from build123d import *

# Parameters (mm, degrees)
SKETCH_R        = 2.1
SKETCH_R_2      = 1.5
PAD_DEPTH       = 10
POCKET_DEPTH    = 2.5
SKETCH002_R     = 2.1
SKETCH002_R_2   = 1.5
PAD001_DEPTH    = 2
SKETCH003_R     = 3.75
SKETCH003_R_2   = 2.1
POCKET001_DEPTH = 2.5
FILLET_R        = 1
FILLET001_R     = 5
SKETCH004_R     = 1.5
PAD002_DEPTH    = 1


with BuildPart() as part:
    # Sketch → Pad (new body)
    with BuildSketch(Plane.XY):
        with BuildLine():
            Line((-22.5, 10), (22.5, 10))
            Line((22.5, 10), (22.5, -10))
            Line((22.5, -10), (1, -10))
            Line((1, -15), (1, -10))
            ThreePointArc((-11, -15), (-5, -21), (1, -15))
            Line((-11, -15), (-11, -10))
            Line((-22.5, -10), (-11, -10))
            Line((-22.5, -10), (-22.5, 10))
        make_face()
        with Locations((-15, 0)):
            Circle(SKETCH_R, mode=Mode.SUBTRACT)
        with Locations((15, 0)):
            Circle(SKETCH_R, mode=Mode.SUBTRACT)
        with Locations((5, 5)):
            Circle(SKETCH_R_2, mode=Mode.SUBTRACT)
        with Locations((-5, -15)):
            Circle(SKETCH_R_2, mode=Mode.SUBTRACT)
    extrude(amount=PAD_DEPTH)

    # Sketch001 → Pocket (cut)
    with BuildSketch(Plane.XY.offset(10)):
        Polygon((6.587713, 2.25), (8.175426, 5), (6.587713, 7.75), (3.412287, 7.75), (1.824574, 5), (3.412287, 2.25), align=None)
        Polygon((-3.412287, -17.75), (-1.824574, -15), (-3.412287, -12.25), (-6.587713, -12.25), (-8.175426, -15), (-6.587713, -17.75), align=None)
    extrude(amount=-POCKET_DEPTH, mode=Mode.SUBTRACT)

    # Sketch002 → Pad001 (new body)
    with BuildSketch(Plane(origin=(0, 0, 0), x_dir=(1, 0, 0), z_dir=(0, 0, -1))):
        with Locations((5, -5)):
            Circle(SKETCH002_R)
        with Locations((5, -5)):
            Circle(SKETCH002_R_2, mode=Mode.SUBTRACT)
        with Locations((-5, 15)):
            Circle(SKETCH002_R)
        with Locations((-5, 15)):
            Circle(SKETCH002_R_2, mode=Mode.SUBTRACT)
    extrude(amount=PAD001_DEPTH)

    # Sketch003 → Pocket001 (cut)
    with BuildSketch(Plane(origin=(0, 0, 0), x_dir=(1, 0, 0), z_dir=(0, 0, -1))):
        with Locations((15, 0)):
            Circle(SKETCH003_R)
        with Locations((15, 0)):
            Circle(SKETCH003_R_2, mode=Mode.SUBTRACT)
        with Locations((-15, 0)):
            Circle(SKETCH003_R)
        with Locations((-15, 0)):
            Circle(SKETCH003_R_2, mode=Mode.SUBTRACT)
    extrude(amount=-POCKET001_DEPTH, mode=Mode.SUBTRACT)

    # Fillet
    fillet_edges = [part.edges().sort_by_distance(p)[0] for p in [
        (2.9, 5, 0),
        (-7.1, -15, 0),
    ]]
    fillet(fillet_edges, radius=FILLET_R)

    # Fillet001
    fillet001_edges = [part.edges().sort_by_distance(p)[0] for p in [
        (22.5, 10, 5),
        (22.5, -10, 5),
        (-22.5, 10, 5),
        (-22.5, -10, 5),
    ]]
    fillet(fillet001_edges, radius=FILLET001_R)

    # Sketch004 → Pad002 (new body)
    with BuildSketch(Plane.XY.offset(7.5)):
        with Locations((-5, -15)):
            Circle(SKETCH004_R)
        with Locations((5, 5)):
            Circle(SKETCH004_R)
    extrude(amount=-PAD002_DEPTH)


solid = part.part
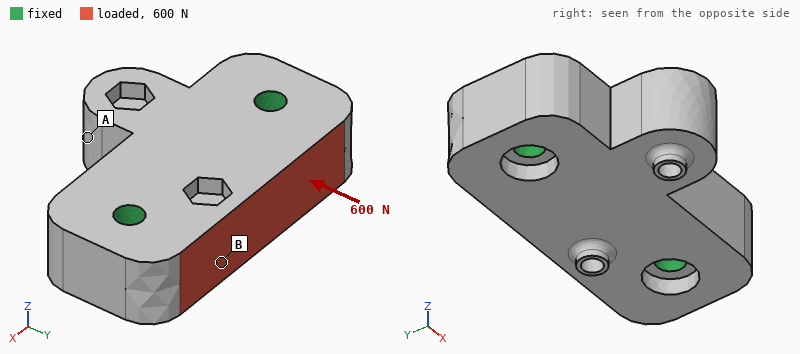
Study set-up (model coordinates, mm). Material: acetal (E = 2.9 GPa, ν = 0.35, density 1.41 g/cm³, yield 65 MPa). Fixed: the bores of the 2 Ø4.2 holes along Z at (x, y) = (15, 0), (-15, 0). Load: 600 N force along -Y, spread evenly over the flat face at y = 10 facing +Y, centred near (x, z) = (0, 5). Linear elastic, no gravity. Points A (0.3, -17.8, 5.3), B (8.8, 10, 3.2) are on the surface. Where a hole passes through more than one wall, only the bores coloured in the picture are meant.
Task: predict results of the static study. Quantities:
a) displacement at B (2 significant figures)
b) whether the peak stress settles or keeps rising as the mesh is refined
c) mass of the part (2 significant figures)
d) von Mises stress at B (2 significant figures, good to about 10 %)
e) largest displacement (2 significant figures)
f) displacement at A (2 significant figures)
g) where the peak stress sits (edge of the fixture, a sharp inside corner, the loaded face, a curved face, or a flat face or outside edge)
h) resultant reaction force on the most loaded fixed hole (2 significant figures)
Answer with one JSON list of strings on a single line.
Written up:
["19 µm", "keeps rising", "13 g", "1.8 MPa", "27 µm", "21 µm", "edge of the fixture", "300 N"]
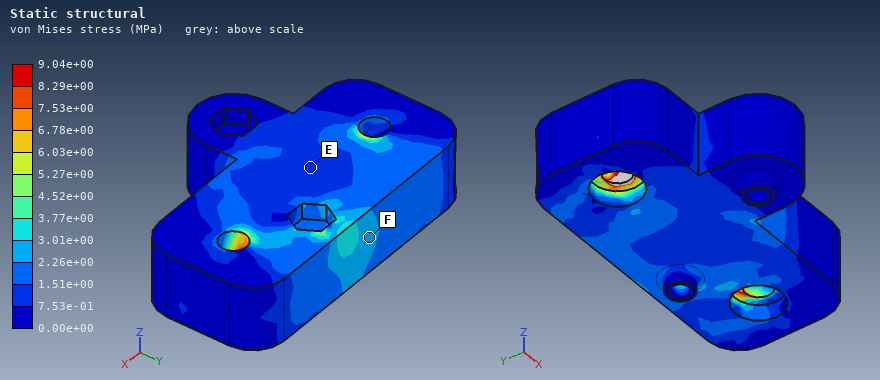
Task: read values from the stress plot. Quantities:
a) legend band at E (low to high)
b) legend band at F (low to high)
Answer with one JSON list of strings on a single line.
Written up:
["7.53e-01 to 1.51e+00 MPa", "2.26e+00 to 3.01e+00 MPa"]
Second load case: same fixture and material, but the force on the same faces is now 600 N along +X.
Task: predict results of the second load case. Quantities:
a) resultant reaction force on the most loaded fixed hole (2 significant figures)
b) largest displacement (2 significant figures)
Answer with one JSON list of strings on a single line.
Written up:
["350 N", "22 µm"]
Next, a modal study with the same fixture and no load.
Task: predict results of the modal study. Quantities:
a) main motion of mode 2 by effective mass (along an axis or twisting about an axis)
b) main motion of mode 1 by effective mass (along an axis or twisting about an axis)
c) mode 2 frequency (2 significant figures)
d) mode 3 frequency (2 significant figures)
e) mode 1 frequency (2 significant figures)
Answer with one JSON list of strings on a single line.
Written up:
["along Z", "along Z", "7900 Hz", "8500 Hz", "4400 Hz"]
